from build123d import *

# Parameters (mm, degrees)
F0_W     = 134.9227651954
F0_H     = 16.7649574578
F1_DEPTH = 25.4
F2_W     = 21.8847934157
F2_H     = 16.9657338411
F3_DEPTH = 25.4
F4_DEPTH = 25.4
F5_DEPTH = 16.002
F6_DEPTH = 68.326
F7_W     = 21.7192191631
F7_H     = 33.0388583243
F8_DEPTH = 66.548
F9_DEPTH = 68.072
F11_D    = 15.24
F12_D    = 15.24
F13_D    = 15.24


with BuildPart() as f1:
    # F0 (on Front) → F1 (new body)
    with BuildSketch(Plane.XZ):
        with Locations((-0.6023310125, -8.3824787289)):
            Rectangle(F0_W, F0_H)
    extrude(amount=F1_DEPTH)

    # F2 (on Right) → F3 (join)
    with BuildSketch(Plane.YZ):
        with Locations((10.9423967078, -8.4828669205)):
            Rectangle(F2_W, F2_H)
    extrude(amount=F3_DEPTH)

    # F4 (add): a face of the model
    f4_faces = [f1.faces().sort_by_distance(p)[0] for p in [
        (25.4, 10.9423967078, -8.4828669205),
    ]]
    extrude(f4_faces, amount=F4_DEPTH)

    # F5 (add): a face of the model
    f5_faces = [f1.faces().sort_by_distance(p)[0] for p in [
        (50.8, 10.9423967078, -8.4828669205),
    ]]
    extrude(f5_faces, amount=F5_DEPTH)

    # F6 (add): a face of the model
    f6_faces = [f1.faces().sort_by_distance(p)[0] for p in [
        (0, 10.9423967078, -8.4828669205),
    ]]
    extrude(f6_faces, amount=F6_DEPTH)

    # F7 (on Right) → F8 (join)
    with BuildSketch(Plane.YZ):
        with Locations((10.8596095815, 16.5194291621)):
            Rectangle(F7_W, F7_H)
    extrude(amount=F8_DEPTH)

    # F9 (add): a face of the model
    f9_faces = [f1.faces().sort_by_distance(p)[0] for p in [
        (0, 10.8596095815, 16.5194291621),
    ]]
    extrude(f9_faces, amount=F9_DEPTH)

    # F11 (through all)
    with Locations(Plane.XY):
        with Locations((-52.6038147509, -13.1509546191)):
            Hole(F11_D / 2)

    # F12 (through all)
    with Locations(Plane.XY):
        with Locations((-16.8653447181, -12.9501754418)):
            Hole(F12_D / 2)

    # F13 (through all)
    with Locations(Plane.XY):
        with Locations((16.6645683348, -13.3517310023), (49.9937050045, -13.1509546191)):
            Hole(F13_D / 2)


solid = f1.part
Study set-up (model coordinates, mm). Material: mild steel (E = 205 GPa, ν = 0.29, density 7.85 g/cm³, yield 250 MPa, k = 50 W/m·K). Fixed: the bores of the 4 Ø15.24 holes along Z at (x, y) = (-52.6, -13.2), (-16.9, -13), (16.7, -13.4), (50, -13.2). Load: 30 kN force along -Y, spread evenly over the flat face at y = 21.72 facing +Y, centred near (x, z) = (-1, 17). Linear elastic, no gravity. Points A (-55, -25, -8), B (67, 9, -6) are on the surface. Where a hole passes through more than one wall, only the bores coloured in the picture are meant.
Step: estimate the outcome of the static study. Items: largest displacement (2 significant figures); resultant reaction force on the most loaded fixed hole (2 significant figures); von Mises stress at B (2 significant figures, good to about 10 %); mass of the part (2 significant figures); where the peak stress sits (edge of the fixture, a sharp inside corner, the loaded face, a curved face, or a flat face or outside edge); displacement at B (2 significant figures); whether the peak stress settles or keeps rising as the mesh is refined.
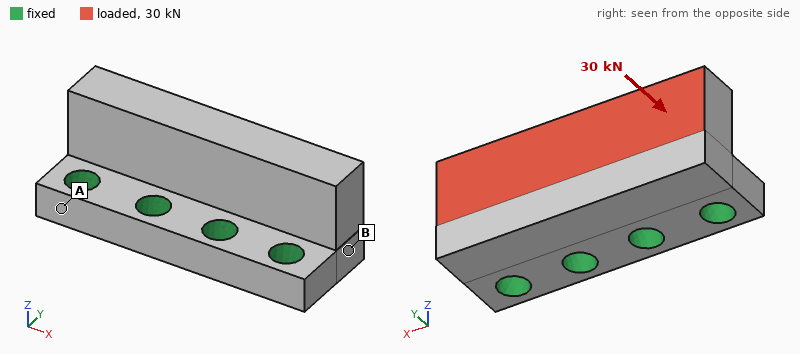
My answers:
61 µm
8.1 kN
38 MPa
1.5 kg
edge of the fixture
11 µm
keeps rising
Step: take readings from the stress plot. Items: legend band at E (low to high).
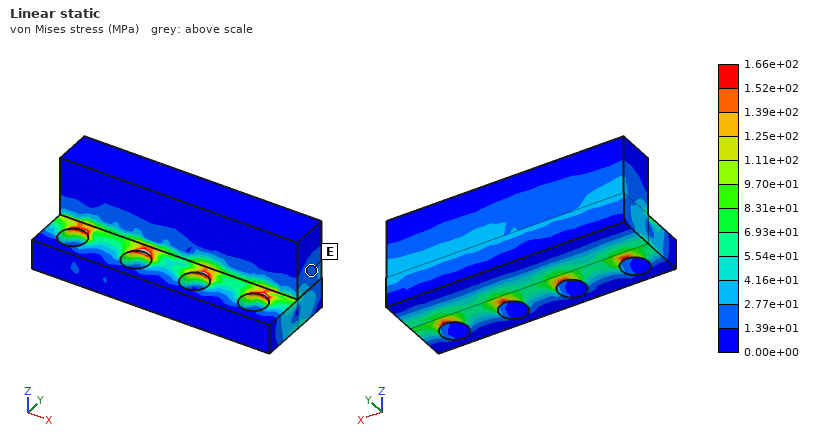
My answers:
1.39e+01 to 2.77e+01 MPa
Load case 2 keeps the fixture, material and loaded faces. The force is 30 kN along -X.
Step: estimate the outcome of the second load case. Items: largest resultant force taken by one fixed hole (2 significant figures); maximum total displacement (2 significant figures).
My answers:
12 kN
13 µm
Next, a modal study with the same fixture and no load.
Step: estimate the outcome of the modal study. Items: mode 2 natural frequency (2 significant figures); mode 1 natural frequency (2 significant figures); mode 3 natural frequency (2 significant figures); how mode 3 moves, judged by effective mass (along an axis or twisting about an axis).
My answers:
6500 Hz
4500 Hz
11 kHz
along X
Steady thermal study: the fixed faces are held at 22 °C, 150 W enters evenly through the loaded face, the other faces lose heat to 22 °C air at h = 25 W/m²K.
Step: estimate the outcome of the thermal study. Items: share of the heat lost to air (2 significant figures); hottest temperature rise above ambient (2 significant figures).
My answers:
7.2 %
44 K
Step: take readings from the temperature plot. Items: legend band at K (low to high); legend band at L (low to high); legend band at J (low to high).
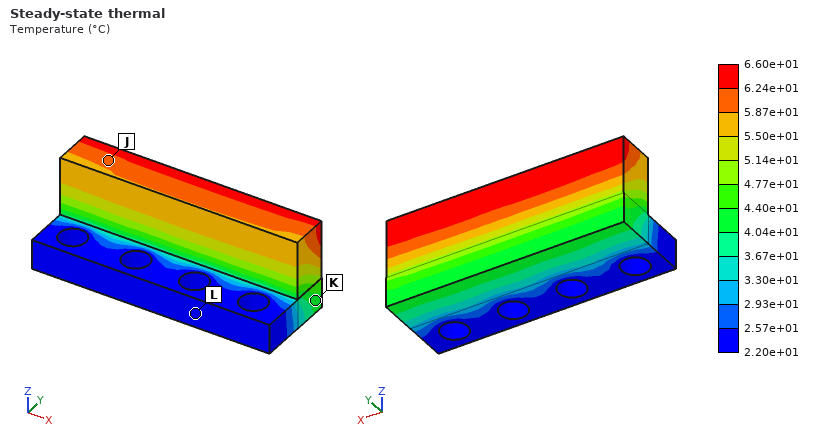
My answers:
4.04e+01 to 4.40e+01 °C
2.20e+01 to 2.57e+01 °C
5.87e+01 to 6.24e+01 °C
